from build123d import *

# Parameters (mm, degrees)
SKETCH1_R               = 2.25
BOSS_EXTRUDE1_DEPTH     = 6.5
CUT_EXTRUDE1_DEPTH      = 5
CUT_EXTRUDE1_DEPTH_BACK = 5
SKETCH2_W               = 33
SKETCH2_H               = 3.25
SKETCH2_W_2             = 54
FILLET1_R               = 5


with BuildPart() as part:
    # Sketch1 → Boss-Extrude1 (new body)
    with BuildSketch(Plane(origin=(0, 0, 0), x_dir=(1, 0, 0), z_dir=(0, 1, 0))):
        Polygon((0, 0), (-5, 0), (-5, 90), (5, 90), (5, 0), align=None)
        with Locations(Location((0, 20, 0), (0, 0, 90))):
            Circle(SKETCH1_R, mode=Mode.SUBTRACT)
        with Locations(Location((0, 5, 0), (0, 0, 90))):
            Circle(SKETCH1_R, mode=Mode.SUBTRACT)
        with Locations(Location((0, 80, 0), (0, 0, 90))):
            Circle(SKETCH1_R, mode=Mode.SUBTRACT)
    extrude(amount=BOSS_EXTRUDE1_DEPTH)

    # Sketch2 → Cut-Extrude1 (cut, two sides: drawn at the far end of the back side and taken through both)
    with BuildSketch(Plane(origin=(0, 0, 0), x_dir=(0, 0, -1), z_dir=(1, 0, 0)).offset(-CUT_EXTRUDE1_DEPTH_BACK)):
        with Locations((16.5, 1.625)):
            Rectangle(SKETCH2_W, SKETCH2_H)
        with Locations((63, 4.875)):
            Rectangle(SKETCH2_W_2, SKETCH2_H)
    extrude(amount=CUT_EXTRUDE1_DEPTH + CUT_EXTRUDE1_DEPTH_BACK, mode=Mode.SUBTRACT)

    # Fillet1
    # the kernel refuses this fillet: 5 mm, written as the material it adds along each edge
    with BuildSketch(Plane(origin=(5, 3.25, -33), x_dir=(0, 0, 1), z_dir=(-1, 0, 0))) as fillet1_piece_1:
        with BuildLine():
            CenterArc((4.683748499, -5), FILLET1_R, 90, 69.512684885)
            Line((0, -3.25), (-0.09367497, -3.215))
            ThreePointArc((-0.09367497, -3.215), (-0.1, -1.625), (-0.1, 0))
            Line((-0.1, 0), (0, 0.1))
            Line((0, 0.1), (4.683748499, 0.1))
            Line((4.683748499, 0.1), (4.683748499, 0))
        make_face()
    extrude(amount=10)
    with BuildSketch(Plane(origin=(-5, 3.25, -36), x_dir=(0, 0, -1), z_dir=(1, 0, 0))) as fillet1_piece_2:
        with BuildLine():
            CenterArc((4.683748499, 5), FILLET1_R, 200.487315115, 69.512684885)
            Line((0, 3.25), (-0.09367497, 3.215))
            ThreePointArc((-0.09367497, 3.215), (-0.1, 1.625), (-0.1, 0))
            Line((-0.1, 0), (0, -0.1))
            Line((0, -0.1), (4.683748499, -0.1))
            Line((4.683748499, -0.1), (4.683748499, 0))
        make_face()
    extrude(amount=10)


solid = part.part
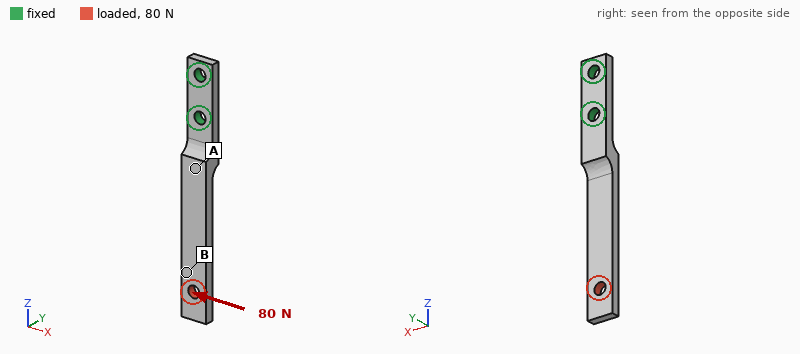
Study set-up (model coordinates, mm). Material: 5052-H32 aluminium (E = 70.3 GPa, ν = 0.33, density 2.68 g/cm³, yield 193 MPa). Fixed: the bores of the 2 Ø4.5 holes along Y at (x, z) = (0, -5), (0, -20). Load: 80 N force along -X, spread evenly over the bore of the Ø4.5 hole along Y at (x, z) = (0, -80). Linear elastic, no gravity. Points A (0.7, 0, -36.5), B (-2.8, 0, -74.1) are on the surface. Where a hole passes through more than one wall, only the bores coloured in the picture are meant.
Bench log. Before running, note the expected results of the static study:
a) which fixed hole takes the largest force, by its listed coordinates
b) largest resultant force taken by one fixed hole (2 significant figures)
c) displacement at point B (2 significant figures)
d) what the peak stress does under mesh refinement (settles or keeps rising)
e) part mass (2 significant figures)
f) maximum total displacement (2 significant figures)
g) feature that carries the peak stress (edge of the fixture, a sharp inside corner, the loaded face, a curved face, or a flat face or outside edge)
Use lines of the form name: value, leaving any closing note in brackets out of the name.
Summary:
which fixed hole takes the largest force, by its listed coordinates: (0, -20)
largest resultant force taken by one fixed hole: 160 N
displacement at point B: 0.28 mm
what the peak stress does under mesh refinement: keeps rising
part mass: 7.9 g
maximum total displacement: 0.40 mm
feature that carries the peak stress: edge of the fixture
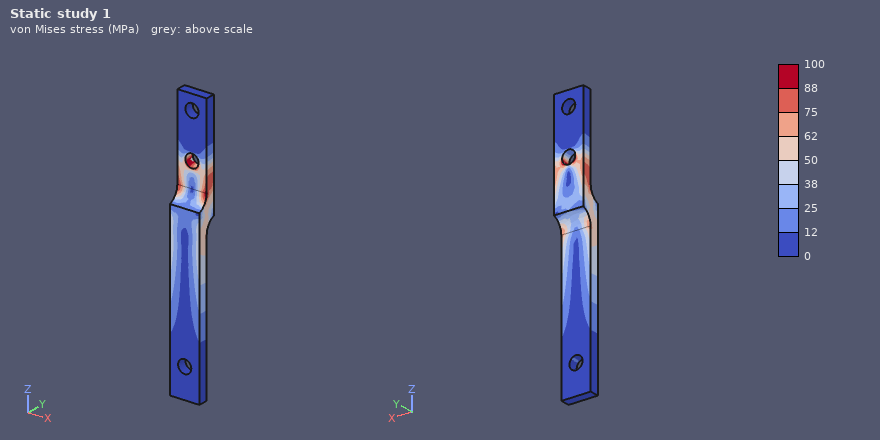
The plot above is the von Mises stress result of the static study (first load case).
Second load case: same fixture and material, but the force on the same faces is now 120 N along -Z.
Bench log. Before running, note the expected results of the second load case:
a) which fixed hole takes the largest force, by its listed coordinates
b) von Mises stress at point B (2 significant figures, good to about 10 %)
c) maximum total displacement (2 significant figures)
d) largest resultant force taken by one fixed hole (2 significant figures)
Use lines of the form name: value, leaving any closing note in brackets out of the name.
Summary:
which fixed hole takes the largest force, by its listed coordinates: (0, -20)
von Mises stress at point B: 3.8 MPa
maximum total displacement: 0.13 mm
largest resultant force taken by one fixed hole: 120 N
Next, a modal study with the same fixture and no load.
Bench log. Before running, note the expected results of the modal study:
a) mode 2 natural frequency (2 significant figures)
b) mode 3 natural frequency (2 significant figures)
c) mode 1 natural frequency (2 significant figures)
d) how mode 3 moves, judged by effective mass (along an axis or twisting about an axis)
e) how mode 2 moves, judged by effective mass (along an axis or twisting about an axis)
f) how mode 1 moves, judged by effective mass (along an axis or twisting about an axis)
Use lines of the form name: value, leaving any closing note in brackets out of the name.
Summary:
mode 2 natural frequency: 1700 Hz
mode 3 natural frequency: 3500 Hz
mode 1 natural frequency: 650 Hz
how mode 3 moves, judged by effective mass: along Y
how mode 2 moves, judged by effective mass: along X
how mode 1 moves, judged by effective mass: along Y
